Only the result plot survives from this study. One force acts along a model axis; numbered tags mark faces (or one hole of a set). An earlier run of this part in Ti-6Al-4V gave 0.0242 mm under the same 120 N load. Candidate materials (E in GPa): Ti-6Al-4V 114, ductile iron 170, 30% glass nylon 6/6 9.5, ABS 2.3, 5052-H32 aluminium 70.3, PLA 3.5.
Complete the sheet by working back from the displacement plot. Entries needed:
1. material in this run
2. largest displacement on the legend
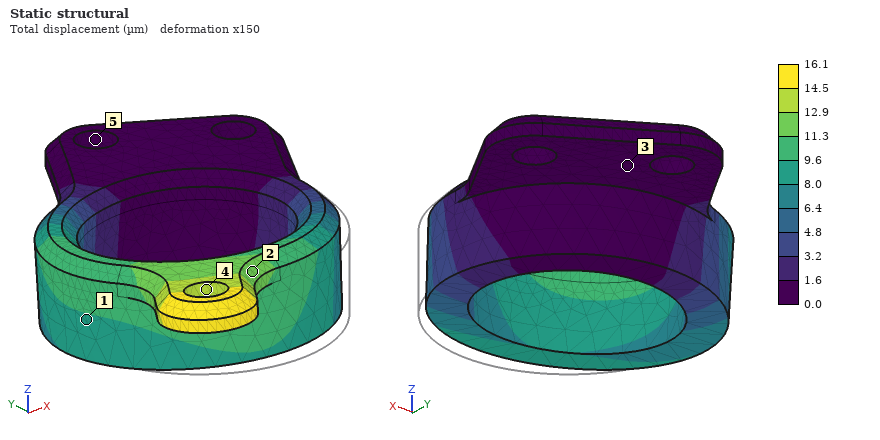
ductile iron
16.1 µm
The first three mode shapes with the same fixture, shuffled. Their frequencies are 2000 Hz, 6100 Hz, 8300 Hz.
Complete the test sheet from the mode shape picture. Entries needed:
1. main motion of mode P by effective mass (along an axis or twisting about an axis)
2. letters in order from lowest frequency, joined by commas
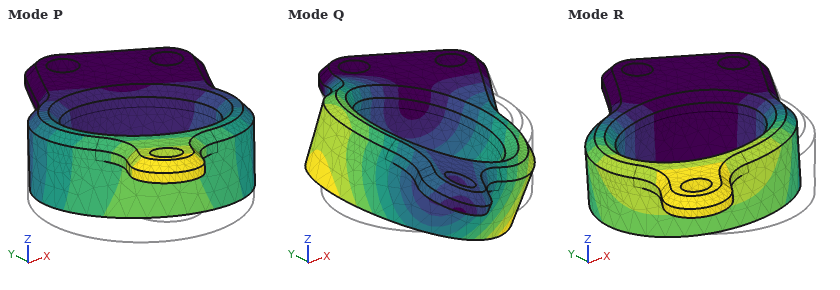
along Z
P, R, Q
